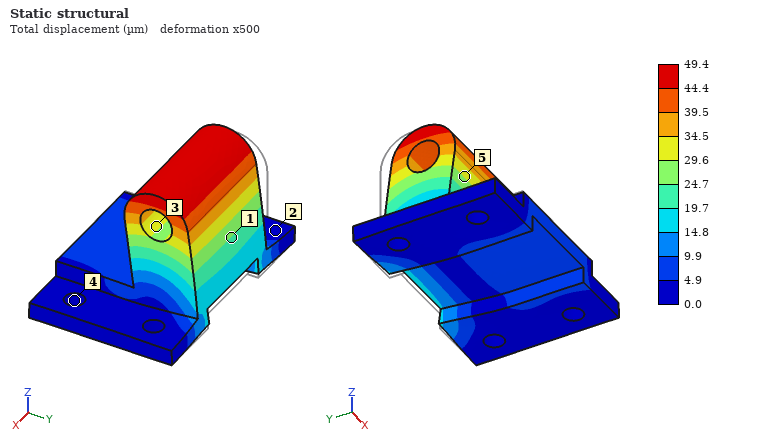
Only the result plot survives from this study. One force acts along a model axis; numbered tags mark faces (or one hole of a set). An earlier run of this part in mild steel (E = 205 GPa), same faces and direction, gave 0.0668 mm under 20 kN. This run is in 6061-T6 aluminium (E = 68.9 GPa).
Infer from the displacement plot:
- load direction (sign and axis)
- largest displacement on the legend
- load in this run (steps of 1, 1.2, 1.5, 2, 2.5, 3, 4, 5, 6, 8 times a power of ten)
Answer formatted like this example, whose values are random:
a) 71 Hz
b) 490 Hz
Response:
a) -Y
b) 49.4 µm
c) 5 kN
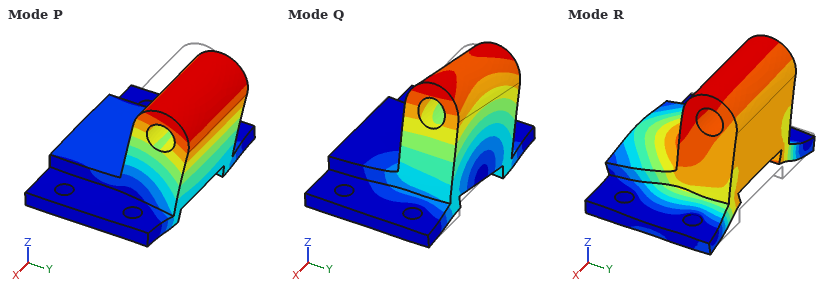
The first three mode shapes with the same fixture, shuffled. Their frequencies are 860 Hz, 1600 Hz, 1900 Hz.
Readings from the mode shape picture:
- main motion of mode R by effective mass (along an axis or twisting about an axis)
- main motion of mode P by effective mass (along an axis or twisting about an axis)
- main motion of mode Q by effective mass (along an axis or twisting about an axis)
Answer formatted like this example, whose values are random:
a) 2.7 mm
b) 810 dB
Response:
a) along Z
b) along Y
c) along X
